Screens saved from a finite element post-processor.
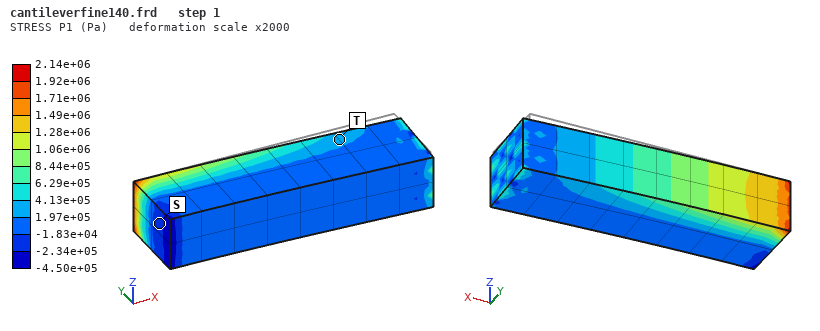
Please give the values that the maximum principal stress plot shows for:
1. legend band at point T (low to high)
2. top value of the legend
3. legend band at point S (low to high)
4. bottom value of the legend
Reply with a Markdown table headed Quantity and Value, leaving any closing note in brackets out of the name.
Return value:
| Quantity | Value |
|---|---|
| legend band at point T | 1.97e+05 to 4.13e+05 Pa |
| top value of the legend | 2.14e+06 Pa |
| legend band at point S | -2.34e+05 to -1.83e+04 Pa |
| bottom value of the legend | -4.50e+05 Pa |
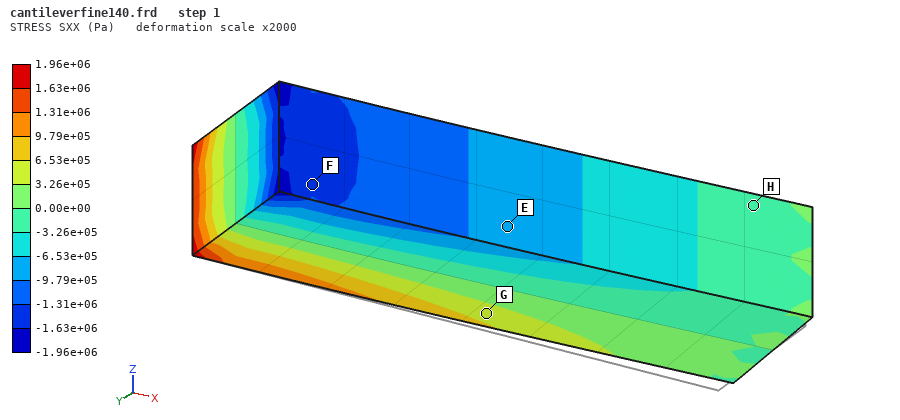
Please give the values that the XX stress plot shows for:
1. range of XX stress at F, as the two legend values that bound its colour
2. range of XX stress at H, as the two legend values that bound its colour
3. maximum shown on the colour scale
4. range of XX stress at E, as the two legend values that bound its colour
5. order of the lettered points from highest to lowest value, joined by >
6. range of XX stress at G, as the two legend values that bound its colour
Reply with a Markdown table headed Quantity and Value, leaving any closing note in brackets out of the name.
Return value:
| Quantity | Value |
|---|---|
| range of XX stress at F, as the two legend values that bound its colour | -1.63e+06 to -1.31e+06 Pa |
| range of XX stress at H, as the two legend values that bound its colour | -3.26e+05 to 0.00e+00 Pa |
| maximum shown on the colour scale | 1.96e+06 Pa |
| range of XX stress at E, as the two legend values that bound its colour | -9.79e+05 to -6.53e+05 Pa |
| order of the lettered points from highest to lowest value, joined by > | G > H > E > F |
| range of XX stress at G, as the two legend values that bound its colour | 3.26e+05 to 6.53e+05 Pa |
